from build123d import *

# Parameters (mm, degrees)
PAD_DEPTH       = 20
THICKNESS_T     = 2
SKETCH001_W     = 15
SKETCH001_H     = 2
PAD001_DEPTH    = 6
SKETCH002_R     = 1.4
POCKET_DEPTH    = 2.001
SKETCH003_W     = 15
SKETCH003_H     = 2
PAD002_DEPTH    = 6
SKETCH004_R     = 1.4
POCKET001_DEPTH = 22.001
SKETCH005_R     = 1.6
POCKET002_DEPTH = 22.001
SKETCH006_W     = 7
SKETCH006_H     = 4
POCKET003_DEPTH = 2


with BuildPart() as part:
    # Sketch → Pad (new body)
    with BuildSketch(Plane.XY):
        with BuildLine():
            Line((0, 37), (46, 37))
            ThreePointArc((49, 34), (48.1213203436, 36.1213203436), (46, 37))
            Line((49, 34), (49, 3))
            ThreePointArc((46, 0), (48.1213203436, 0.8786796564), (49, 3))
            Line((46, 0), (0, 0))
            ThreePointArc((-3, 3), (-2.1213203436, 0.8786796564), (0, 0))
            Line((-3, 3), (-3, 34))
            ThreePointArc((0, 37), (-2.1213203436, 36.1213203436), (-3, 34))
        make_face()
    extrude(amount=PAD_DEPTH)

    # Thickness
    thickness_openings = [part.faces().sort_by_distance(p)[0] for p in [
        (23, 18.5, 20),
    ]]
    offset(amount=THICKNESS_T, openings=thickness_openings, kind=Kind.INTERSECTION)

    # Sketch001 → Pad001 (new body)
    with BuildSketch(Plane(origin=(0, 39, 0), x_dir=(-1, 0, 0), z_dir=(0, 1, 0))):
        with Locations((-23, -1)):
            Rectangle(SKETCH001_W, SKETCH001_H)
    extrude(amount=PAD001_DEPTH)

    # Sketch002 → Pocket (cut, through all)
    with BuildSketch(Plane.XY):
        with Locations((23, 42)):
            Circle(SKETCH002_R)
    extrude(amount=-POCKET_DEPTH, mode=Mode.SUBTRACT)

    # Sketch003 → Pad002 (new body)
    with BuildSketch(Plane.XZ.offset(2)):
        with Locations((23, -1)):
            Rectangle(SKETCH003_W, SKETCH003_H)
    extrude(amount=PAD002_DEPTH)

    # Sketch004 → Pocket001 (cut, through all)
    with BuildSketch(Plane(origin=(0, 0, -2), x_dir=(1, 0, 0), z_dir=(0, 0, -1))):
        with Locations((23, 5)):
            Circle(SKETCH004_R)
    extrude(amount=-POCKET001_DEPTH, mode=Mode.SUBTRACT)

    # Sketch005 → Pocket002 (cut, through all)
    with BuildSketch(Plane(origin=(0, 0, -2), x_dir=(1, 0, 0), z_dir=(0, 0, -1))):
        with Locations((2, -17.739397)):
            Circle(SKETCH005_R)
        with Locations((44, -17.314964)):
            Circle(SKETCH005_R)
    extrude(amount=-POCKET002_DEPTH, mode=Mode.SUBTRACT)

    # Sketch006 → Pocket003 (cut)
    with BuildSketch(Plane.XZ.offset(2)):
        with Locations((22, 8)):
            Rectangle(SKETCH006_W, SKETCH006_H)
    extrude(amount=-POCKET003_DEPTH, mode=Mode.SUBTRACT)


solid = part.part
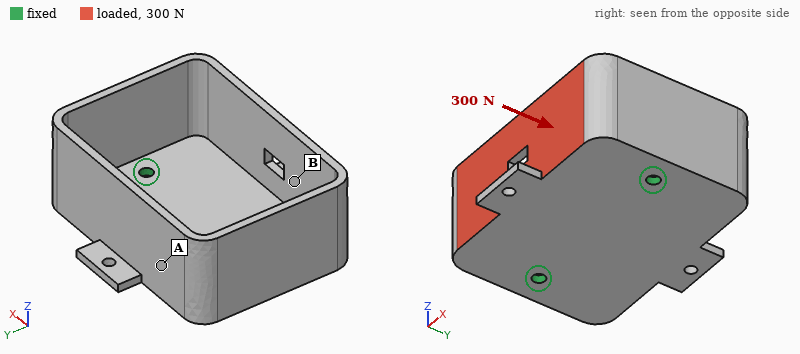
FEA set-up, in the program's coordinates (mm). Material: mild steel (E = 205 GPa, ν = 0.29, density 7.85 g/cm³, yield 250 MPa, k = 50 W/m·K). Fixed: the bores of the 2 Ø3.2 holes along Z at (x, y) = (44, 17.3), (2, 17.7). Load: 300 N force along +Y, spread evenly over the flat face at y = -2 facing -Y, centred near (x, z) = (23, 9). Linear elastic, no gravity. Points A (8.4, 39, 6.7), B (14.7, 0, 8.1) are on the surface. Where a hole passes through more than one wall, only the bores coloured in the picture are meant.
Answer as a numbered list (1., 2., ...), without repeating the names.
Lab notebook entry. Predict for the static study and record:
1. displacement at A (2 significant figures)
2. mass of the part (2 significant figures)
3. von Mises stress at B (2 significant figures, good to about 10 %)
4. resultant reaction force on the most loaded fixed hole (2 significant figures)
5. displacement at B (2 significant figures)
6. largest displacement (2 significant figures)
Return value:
1. 28 µm
2. 94 g
3. 20 MPa
4. 160 N
5. 33 µm
6. 71 µm
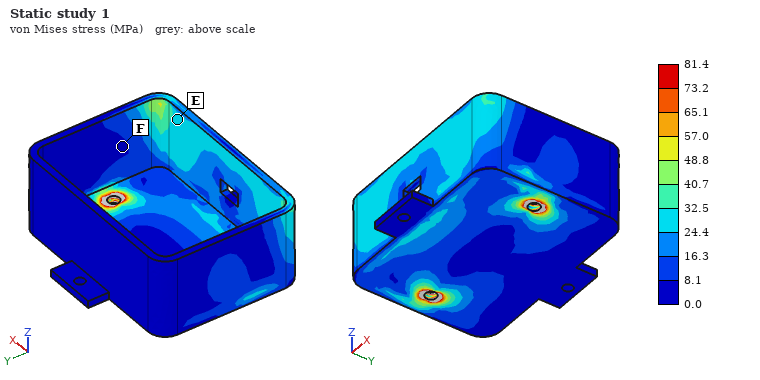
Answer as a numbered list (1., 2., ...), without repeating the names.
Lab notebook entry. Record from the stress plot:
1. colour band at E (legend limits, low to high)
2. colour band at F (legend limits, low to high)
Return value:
1. 24.4 to 32.5 MPa
2. 0.0 to 8.1 MPa
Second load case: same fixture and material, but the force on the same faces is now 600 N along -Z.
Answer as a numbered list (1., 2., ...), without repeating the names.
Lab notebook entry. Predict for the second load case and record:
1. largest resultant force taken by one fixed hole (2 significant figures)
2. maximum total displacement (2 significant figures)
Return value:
1. 310 N
2. 0.15 mm
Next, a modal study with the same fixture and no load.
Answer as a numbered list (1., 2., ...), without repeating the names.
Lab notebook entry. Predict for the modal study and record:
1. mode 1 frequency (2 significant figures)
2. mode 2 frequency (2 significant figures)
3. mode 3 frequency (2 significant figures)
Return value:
1. 1500 Hz
2. 2500 Hz
3. 4500 Hz
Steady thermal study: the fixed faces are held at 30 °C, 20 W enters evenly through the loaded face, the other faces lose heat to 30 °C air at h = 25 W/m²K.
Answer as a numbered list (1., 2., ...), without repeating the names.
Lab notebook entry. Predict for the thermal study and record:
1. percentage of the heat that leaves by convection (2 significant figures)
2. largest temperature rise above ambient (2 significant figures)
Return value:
1. 36 %
2. 78 K
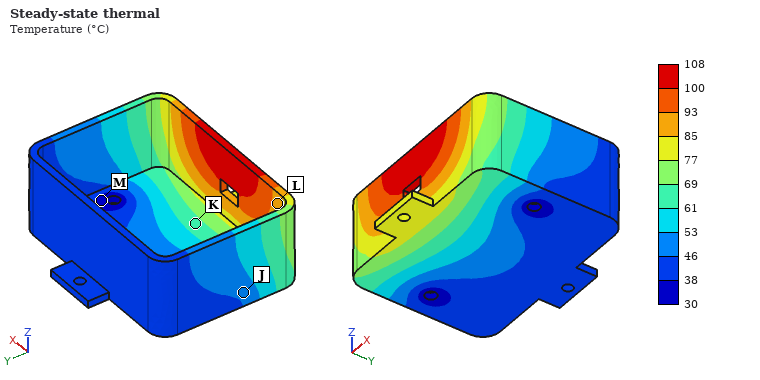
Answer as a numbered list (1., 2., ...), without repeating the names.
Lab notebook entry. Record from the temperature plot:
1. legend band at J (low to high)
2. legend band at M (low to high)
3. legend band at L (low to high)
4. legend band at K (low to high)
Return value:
1. 46 to 53 °C
2. 30 to 38 °C
3. 85 to 93 °C
4. 61 to 69 °C
